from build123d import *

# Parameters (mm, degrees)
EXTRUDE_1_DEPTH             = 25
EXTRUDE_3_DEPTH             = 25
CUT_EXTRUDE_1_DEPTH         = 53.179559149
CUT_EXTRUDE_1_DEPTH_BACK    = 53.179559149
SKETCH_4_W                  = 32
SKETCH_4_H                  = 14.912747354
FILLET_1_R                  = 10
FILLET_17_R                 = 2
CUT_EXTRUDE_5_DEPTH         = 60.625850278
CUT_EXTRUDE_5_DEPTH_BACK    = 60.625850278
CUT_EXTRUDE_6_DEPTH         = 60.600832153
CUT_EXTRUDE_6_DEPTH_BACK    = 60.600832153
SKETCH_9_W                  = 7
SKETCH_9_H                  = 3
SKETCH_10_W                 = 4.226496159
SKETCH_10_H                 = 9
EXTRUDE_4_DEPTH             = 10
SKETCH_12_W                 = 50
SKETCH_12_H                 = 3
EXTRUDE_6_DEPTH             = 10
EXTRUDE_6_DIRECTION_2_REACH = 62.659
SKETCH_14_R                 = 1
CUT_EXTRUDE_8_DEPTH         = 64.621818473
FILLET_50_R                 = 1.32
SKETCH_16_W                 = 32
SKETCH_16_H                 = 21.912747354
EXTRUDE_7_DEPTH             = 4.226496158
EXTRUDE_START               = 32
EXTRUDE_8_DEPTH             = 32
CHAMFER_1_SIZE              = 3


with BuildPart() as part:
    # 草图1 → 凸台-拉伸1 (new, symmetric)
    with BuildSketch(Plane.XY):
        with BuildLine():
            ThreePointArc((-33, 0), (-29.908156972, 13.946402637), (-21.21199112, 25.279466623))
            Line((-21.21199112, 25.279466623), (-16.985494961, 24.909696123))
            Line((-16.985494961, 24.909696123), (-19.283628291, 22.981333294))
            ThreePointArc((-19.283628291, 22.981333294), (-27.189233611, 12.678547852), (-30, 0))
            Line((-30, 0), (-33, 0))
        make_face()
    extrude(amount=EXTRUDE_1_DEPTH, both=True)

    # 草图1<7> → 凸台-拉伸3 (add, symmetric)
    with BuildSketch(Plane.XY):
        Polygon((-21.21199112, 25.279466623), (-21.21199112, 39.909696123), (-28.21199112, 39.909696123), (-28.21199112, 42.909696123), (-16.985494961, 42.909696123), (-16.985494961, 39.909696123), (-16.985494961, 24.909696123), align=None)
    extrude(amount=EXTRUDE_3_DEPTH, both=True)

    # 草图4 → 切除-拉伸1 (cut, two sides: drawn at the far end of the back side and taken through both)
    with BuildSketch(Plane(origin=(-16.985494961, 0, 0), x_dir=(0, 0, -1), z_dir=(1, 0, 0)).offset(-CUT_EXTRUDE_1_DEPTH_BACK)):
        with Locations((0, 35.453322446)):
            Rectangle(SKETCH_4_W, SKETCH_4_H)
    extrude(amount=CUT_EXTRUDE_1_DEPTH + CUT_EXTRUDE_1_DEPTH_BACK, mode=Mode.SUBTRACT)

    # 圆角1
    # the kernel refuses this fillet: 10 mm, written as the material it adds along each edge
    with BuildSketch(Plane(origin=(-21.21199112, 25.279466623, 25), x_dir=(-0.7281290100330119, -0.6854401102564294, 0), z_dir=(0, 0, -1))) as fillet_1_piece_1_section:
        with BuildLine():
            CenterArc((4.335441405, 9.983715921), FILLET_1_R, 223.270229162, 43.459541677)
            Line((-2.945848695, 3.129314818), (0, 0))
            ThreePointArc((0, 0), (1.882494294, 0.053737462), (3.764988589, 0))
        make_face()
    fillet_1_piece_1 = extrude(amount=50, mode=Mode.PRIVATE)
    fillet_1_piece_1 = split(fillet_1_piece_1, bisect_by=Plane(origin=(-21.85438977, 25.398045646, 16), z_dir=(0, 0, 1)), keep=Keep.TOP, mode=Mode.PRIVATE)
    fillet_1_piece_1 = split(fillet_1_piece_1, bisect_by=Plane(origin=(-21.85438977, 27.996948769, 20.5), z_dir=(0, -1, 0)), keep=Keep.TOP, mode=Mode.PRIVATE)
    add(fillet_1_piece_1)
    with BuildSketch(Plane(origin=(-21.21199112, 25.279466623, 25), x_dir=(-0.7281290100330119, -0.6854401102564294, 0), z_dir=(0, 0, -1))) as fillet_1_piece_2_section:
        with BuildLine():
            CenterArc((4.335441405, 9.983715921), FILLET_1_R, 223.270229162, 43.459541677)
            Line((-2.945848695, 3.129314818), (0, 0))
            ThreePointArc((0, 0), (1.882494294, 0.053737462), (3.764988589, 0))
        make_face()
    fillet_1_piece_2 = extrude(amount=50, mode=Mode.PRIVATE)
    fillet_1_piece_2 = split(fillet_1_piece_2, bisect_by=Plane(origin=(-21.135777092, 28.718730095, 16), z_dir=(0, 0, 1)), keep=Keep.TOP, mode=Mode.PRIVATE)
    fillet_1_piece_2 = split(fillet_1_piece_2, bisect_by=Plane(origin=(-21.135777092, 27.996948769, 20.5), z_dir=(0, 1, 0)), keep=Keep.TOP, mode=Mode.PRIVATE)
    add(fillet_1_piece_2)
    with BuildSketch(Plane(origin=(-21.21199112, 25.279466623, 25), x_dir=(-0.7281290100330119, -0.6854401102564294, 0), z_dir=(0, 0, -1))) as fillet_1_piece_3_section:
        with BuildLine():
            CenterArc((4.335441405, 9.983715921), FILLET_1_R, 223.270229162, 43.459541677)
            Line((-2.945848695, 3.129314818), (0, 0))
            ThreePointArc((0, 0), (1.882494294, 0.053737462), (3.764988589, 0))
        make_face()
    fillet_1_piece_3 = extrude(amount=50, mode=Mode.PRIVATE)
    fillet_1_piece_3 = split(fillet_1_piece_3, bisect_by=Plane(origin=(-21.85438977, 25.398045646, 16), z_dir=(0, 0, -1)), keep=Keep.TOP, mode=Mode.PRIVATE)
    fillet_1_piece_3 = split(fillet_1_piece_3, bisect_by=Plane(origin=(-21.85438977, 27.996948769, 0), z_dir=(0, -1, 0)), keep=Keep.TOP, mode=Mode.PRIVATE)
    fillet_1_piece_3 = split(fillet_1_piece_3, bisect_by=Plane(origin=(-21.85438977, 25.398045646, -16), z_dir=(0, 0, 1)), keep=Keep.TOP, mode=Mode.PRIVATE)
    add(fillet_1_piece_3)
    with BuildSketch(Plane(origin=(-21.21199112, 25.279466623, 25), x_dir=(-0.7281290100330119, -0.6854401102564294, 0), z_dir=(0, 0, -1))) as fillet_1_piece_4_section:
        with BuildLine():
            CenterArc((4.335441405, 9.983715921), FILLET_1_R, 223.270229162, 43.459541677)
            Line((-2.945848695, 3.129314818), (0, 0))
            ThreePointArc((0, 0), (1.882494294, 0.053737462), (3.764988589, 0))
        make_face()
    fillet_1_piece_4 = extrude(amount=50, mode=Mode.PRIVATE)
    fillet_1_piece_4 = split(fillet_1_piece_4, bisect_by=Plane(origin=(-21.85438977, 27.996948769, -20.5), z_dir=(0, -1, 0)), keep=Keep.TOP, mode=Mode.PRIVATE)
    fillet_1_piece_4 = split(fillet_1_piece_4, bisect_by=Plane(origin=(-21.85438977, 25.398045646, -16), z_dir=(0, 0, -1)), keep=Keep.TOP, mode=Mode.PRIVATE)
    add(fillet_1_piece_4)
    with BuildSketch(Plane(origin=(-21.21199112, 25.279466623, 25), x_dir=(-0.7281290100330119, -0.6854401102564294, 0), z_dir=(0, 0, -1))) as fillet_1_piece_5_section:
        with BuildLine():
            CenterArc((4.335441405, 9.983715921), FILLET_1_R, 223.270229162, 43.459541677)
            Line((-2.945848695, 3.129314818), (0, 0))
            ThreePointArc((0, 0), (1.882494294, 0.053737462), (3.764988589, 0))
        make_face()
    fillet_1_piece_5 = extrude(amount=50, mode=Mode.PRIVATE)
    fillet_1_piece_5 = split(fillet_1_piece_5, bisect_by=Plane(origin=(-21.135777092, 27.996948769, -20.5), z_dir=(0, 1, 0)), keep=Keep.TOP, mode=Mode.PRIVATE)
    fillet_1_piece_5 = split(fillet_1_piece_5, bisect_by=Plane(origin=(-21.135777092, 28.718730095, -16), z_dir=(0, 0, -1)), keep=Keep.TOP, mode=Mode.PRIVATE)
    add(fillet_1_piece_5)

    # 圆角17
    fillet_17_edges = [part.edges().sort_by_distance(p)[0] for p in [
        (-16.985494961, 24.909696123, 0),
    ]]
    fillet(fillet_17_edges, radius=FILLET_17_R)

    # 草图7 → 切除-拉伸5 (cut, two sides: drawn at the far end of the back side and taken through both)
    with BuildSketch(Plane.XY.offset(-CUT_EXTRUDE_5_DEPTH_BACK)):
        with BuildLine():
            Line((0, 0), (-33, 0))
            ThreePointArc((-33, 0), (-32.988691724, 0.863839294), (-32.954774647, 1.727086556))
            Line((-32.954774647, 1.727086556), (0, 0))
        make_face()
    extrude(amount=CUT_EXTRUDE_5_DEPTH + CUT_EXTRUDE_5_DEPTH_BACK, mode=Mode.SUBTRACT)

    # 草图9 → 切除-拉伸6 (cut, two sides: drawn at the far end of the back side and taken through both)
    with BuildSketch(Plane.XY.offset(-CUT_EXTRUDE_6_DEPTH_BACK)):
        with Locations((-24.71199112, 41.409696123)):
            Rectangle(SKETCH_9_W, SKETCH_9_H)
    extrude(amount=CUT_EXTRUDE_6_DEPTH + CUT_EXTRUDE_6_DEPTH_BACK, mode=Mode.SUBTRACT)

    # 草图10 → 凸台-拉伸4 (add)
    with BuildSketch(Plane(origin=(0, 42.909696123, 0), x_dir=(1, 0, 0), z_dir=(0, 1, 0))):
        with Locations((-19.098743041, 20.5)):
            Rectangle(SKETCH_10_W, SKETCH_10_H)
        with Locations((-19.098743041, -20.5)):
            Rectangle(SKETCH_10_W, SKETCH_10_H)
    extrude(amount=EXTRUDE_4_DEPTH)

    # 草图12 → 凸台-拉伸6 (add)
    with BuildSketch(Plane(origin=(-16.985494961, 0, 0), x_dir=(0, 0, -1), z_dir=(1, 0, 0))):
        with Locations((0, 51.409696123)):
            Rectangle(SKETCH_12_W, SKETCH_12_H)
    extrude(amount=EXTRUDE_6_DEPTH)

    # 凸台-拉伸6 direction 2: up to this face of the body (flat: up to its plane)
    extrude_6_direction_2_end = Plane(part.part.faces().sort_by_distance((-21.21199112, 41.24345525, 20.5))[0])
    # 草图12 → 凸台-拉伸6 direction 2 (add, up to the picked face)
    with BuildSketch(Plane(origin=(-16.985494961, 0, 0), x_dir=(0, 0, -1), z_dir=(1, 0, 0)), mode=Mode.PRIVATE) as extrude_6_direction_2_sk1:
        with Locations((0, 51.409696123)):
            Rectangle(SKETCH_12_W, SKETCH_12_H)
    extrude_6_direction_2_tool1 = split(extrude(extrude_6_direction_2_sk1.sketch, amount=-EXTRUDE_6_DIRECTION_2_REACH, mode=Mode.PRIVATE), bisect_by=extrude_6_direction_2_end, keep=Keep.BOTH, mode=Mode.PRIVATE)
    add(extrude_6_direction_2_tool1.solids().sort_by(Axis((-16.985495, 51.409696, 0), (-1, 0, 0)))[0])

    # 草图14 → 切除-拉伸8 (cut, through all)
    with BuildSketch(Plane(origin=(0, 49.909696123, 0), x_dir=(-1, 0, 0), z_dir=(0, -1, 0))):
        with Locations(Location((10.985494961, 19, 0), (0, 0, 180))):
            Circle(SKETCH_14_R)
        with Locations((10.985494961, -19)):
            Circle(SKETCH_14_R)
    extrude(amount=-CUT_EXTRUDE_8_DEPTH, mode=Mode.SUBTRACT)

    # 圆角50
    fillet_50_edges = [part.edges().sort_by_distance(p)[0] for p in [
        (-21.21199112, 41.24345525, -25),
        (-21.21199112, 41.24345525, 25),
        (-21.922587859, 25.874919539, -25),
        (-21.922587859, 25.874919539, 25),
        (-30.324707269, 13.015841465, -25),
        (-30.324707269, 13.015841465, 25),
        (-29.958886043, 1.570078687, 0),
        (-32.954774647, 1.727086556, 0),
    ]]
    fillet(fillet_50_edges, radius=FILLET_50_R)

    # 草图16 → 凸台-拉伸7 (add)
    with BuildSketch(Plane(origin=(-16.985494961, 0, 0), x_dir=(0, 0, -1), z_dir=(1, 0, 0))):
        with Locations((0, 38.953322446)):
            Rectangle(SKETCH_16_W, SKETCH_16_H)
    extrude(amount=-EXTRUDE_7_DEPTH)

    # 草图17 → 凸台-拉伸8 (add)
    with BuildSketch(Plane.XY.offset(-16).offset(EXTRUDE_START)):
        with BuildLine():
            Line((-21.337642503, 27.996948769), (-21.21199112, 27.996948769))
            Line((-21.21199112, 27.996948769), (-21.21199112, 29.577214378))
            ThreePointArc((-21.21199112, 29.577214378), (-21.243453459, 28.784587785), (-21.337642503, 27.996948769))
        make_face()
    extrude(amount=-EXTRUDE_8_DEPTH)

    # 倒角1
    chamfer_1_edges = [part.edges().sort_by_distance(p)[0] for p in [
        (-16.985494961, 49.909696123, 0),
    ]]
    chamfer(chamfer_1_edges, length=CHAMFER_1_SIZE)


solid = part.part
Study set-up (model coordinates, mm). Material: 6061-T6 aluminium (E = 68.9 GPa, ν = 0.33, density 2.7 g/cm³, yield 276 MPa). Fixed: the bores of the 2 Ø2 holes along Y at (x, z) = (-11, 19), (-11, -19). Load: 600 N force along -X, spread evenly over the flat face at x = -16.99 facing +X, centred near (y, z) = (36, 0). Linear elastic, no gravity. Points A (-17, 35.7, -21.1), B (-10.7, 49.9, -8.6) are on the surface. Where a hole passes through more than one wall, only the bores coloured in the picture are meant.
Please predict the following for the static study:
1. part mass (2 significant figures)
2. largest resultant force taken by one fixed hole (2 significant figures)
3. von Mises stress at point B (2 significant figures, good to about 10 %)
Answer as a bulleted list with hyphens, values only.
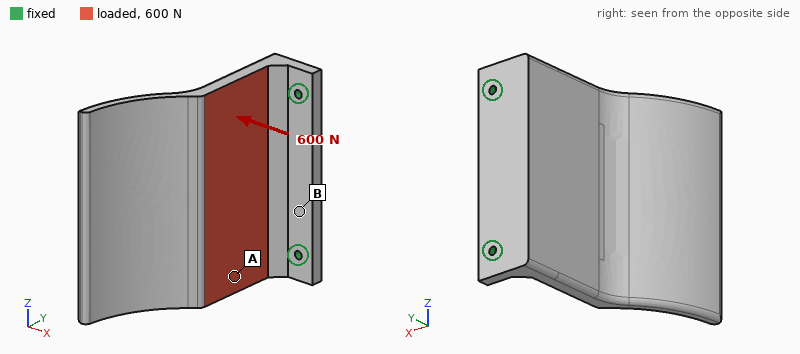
- 32 g
- 330 N
- 59 MPa
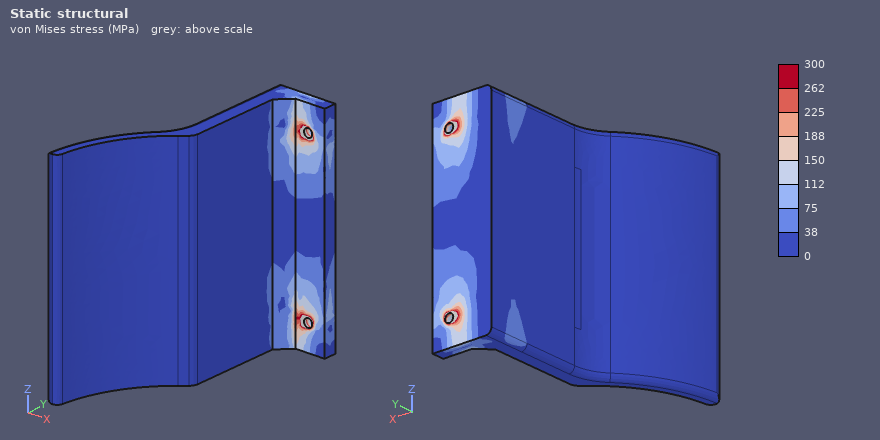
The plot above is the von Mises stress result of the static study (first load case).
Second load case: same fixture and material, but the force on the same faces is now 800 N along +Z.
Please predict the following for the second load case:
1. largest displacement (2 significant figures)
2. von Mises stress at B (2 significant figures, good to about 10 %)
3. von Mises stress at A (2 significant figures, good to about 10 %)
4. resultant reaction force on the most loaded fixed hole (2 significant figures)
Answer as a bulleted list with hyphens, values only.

- 54 µm
- 14 MPa
- 13 MPa
- 520 N
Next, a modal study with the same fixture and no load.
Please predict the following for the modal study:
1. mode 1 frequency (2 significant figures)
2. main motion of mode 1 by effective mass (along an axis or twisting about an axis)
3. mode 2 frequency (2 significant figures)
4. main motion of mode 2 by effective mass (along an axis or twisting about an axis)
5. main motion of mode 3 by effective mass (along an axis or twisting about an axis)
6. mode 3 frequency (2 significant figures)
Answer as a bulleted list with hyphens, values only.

- 830 Hz
- along X
- 2800 Hz
- twisting about Y
- along Z
- 4700 Hz
